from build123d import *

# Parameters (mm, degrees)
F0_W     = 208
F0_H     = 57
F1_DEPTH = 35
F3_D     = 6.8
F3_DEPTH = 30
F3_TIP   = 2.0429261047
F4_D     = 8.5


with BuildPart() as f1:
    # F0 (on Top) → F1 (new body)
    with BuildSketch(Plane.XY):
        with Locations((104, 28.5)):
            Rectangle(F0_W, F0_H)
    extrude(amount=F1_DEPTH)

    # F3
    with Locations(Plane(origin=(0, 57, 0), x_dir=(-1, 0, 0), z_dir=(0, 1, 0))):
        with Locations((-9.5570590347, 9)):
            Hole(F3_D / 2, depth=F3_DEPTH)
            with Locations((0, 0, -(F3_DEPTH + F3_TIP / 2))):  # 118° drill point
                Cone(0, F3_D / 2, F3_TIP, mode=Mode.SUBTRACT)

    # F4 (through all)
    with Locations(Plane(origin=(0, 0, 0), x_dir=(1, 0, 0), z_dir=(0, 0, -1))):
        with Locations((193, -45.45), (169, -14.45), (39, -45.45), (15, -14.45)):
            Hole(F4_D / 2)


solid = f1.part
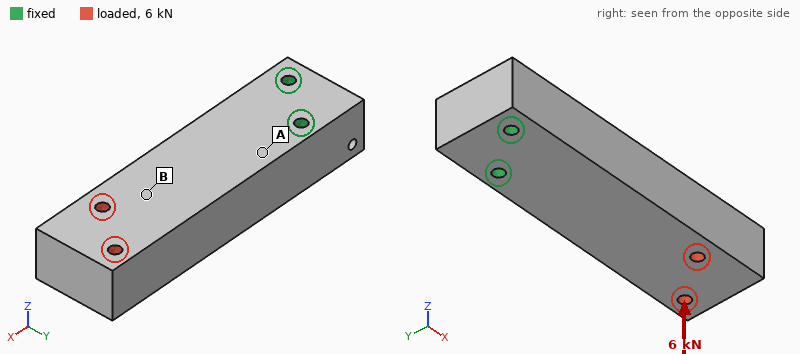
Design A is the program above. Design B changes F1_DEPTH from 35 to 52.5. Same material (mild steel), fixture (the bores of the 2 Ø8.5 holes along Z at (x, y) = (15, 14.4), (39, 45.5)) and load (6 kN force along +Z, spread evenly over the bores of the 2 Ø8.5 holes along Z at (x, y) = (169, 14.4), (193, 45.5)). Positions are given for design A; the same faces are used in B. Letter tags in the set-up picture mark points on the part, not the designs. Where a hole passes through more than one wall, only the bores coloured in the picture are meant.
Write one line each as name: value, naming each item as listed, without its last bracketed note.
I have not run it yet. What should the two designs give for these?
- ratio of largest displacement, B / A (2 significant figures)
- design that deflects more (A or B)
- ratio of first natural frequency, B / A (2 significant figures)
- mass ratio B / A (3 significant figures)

ratio of largest displacement, B / A: 0.32
design that deflects more: A
ratio of first natural frequency, B / A: 1.4
mass ratio B / A: 1.50
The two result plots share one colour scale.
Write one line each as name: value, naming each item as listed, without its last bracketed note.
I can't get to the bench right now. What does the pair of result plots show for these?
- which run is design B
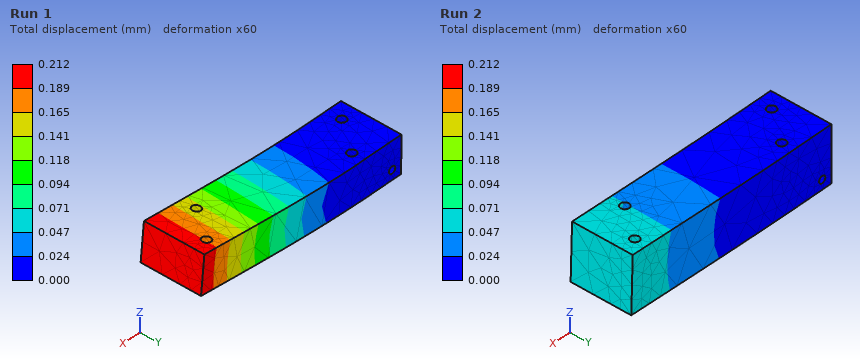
which run is design B: Run 2
